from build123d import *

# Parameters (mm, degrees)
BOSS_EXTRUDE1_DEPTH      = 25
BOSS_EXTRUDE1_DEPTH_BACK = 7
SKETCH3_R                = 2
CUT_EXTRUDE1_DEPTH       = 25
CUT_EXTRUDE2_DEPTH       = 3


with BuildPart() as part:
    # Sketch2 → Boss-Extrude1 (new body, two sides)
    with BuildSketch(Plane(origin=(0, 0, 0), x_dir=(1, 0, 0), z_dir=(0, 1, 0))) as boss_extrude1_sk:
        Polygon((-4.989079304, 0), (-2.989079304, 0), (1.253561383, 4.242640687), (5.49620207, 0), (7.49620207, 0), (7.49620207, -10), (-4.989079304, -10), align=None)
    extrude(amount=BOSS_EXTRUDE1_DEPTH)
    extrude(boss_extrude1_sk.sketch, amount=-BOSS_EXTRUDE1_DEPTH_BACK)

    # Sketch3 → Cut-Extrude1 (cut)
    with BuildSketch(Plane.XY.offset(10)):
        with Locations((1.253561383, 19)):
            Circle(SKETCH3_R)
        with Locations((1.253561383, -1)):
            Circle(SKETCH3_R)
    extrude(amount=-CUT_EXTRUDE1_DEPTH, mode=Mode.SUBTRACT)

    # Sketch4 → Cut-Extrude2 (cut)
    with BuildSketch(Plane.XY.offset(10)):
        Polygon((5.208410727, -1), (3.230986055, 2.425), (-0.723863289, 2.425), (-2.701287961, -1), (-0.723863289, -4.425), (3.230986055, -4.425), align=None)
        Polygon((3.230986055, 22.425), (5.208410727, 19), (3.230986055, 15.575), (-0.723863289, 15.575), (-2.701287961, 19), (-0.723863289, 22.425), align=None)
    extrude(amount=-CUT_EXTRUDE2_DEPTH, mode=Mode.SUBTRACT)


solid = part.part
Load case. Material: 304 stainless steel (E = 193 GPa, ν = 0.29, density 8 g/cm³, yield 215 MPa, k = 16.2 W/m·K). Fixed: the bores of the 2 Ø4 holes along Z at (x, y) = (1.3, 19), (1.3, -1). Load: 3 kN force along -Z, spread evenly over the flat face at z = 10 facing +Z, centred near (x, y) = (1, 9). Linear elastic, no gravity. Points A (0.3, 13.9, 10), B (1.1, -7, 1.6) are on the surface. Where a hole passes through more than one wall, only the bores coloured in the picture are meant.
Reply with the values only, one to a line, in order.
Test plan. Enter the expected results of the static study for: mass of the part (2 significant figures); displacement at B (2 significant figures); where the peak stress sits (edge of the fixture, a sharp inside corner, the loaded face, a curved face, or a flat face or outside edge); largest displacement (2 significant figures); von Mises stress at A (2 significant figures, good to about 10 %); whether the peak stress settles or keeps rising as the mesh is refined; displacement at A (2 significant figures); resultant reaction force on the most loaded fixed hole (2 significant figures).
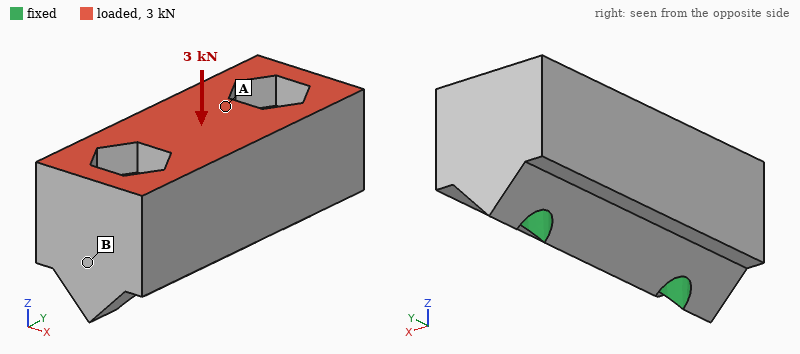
33 g
0.21 µm
edge of the fixture
1.1 µm
12 MPa
keeps rising
0.81 µm
1.5 kN
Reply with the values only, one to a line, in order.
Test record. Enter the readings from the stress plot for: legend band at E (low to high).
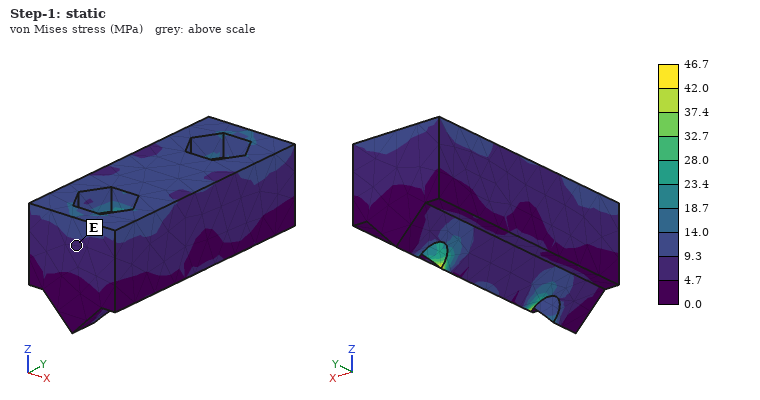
4.7 to 9.3 MPa
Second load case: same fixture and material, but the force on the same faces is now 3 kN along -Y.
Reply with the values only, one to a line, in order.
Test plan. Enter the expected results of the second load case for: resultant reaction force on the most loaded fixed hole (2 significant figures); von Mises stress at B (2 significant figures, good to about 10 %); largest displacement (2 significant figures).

1.7 kN
7.5 MPa
2.3 µm
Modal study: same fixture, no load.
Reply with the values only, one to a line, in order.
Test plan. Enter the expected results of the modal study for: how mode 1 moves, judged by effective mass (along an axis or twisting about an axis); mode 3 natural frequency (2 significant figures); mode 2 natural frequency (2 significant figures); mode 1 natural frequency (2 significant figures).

along X
63 kHz
62 kHz
49 kHz
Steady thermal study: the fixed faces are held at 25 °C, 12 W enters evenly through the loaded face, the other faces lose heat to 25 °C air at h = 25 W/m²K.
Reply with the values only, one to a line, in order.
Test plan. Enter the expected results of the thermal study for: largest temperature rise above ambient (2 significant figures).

22 K
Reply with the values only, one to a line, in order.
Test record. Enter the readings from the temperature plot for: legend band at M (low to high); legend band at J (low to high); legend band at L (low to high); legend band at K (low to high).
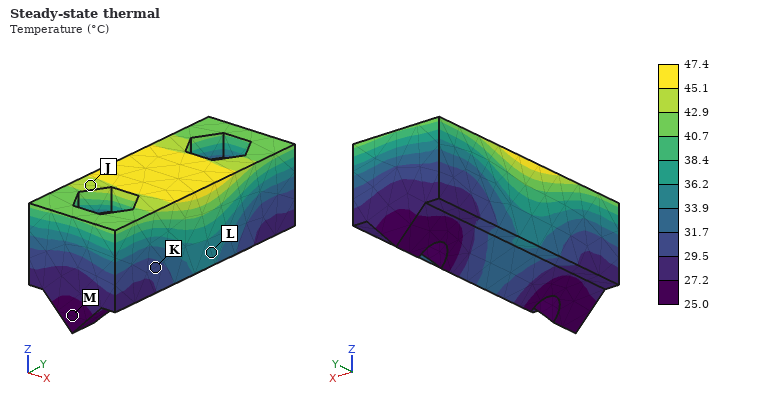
25.0 to 27.2 °C
42.9 to 45.1 °C
33.9 to 36.2 °C
29.5 to 31.7 °C
